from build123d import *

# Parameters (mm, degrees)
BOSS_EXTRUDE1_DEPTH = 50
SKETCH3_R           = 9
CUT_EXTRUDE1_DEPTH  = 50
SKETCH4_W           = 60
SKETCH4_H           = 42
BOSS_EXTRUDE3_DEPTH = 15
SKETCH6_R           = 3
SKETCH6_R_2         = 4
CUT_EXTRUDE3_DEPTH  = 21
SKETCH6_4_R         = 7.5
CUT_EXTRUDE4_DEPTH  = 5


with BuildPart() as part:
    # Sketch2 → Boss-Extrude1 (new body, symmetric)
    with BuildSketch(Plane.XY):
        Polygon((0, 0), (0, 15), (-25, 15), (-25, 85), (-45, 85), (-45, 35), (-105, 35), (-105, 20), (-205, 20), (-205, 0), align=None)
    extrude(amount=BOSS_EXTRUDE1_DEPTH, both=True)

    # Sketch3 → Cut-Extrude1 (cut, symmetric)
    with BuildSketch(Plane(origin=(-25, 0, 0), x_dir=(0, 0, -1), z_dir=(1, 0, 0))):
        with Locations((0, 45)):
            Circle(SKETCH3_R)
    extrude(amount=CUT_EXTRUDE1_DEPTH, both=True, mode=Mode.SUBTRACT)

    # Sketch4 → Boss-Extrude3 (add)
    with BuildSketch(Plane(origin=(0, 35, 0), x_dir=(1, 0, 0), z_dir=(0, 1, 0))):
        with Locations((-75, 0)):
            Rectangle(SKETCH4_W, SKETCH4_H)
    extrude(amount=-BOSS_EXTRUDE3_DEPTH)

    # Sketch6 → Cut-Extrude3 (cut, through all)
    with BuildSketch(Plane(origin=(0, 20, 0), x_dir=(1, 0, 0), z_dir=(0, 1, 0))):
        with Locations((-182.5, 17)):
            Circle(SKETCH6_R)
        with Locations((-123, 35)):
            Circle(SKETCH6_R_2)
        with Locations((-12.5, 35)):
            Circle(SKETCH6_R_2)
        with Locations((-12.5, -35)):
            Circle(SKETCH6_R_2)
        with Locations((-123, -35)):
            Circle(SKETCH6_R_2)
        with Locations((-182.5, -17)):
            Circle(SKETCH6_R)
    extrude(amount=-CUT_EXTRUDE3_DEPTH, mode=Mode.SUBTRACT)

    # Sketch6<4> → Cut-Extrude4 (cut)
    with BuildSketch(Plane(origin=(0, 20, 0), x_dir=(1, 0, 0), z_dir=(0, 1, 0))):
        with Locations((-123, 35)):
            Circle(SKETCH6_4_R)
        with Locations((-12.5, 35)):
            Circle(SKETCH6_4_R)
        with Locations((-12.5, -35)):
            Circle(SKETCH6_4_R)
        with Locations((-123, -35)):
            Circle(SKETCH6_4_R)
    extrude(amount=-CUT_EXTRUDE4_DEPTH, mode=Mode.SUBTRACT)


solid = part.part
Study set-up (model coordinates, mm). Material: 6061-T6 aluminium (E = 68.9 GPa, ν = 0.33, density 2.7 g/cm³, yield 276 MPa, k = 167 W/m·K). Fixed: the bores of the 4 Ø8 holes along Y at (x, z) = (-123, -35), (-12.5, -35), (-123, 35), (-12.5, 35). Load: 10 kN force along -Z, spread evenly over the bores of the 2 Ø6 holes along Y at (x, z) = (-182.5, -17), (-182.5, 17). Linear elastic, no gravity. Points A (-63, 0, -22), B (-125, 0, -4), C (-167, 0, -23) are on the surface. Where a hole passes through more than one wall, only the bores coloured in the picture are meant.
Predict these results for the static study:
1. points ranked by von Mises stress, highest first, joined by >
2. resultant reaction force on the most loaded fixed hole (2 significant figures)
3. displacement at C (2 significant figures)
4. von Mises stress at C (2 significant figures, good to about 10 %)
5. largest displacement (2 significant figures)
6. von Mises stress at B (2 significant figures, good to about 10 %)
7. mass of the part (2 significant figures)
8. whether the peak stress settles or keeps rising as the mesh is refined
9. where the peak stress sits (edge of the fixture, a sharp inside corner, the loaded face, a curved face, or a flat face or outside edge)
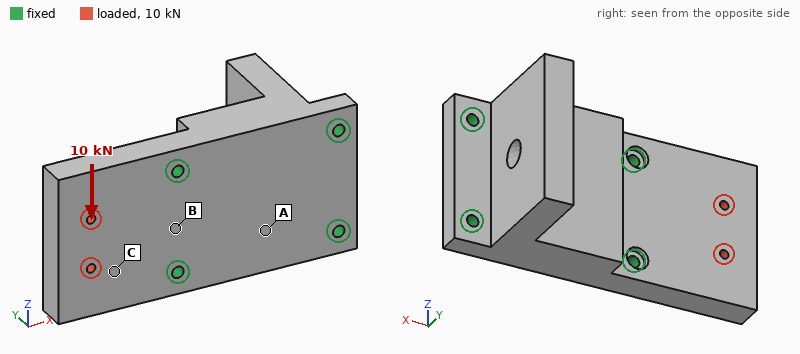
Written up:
C > B > A
8.7 kN
17 µm
11 MPa
31 µm
6.0 MPa
1.6 kg
keeps rising
edge of the fixture
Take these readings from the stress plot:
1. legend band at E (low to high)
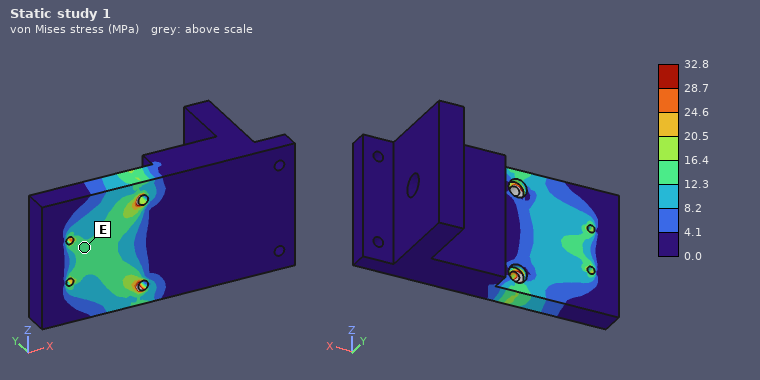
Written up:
12.3 to 16.4 MPa
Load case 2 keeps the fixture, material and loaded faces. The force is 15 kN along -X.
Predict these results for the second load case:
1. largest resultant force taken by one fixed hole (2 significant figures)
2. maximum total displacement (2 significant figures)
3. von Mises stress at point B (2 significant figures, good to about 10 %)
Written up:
6.5 kN
14 µm
3.2 MPa
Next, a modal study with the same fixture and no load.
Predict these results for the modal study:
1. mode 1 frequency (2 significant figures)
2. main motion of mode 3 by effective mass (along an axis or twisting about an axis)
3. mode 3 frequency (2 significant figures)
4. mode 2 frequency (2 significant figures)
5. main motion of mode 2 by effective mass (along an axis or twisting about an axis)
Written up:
1900 Hz
along Z
4100 Hz
3600 Hz
along X
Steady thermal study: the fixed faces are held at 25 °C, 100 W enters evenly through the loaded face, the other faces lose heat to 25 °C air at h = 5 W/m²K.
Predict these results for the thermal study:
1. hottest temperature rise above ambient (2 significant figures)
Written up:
24 K
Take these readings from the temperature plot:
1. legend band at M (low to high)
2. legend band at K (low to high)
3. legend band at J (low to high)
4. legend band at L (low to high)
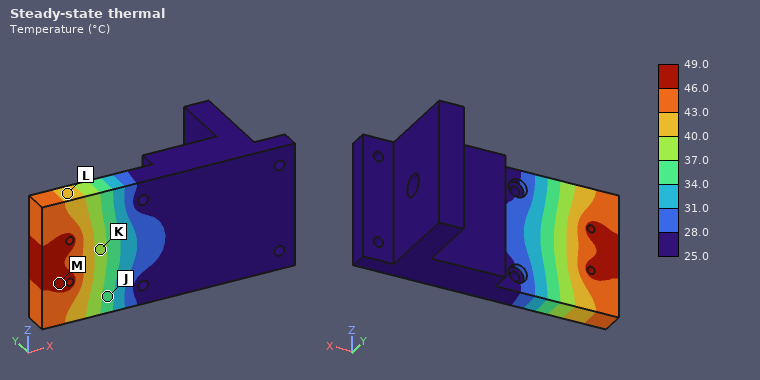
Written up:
46.0 to 49.0 °C
37.0 to 40.0 °C
34.0 to 37.0 °C
40.0 to 43.0 °C
